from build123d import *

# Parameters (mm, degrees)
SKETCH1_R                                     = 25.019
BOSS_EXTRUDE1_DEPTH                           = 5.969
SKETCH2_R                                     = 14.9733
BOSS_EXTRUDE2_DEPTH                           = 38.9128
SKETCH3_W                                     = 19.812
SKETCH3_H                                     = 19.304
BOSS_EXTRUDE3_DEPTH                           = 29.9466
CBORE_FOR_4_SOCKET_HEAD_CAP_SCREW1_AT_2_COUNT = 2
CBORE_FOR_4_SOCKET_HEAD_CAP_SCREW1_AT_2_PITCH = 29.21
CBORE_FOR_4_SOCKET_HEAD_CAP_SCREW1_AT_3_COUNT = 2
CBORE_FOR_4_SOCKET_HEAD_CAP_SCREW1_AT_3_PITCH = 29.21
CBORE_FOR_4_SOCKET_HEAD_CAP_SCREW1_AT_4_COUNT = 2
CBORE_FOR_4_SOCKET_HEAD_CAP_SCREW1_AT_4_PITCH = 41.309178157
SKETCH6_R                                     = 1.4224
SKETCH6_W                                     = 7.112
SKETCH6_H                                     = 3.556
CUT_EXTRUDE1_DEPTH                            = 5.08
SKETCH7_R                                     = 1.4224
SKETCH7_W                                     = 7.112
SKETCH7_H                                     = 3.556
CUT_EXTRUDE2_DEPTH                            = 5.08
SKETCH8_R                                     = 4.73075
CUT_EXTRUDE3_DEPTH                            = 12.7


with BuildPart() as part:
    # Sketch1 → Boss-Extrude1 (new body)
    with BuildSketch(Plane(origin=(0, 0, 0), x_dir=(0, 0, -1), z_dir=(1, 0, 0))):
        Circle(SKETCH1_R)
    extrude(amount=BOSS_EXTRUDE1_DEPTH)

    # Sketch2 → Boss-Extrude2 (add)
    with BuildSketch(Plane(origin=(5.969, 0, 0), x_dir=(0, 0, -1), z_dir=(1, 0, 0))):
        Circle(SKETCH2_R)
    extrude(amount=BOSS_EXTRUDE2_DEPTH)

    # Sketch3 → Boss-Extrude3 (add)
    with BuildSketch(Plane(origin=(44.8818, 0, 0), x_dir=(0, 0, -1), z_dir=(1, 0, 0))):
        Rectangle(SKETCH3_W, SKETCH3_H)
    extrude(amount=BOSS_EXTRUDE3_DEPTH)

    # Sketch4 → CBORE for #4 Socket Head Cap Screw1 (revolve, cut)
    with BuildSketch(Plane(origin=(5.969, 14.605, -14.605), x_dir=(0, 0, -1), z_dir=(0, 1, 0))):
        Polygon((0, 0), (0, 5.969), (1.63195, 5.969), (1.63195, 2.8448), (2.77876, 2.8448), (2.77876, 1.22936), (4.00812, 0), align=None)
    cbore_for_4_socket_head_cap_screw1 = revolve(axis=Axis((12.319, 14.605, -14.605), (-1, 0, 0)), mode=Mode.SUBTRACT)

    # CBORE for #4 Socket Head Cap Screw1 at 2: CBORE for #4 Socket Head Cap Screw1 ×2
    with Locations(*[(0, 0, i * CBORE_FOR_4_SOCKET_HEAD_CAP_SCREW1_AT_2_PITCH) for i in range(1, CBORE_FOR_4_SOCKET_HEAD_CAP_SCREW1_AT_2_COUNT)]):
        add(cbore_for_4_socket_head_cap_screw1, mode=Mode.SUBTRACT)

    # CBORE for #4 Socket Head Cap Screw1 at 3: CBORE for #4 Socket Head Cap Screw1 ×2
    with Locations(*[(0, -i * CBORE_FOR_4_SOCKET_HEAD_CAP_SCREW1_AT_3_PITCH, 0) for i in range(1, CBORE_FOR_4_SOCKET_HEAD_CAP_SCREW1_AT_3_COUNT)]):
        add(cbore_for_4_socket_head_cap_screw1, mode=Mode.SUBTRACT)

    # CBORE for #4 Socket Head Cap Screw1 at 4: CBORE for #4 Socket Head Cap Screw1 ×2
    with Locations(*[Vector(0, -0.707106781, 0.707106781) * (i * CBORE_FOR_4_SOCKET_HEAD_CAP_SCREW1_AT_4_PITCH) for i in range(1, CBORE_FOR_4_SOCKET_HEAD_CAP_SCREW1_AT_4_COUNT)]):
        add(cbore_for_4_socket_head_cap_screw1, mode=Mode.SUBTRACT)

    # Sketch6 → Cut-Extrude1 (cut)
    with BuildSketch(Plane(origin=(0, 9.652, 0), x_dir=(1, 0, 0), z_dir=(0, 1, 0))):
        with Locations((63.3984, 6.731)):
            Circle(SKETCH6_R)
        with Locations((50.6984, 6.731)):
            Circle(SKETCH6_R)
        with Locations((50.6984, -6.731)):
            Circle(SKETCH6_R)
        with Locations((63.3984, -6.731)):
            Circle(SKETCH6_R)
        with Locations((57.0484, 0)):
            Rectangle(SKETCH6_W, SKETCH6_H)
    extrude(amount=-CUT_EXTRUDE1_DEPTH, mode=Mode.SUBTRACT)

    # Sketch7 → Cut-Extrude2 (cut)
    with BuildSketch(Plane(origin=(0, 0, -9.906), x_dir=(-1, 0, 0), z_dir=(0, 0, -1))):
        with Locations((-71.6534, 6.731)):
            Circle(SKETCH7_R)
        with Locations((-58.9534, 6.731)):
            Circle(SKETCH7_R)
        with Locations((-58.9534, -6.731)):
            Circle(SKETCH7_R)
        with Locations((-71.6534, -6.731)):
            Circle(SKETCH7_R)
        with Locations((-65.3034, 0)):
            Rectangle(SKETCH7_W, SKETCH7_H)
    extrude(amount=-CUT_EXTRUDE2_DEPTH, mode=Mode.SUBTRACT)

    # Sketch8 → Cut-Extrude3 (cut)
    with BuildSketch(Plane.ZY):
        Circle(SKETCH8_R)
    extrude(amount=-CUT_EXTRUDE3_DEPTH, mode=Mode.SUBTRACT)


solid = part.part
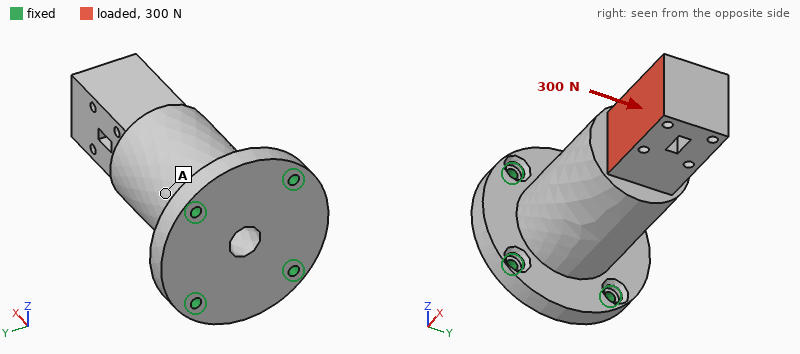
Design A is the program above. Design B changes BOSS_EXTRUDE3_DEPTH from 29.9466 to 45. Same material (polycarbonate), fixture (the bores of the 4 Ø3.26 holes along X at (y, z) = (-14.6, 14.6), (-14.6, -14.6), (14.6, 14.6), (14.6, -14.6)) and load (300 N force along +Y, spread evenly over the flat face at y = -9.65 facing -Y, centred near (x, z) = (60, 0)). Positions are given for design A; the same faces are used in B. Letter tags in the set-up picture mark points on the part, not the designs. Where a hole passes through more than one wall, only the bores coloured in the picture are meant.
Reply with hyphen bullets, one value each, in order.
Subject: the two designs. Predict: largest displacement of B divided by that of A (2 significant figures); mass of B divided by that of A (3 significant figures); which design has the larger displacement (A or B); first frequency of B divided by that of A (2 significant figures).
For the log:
- 1.5
- 1.12
- B
- 0.74
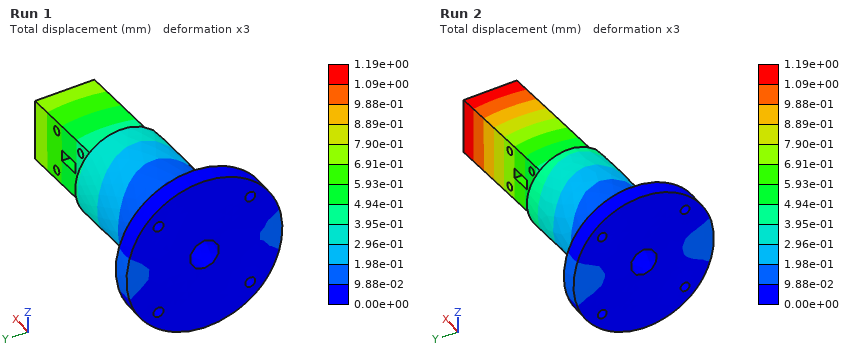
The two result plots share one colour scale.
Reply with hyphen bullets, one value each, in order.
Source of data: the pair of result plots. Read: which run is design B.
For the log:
- Run 2
